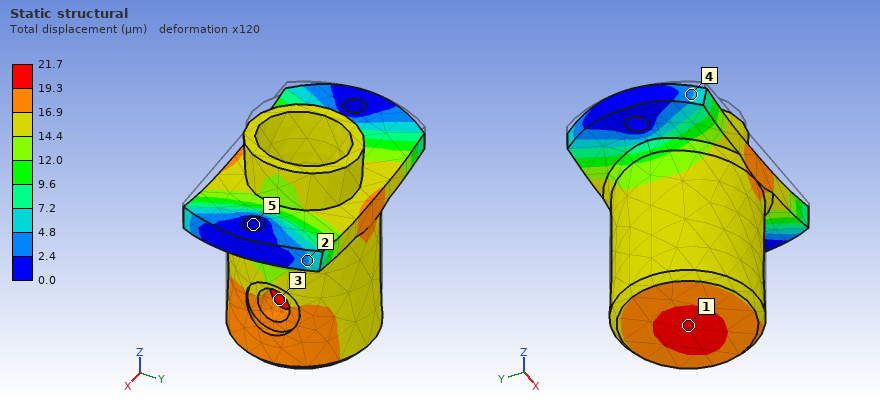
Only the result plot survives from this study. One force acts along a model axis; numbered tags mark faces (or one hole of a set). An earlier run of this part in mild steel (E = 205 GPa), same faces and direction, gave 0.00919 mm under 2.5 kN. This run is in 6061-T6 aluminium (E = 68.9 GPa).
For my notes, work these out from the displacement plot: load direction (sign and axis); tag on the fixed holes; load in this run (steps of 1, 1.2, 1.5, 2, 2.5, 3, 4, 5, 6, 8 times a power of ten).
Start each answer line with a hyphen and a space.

- -Z
- 5
- 2 kN
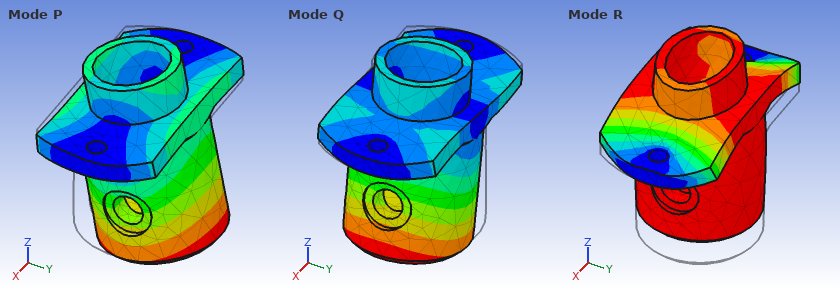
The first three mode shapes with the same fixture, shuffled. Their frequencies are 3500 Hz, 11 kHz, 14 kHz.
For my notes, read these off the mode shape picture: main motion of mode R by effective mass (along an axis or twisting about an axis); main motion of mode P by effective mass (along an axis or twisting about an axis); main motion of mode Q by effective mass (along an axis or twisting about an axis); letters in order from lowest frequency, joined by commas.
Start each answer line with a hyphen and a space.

- along Z
- along Y
- along X
- P, Q, R
